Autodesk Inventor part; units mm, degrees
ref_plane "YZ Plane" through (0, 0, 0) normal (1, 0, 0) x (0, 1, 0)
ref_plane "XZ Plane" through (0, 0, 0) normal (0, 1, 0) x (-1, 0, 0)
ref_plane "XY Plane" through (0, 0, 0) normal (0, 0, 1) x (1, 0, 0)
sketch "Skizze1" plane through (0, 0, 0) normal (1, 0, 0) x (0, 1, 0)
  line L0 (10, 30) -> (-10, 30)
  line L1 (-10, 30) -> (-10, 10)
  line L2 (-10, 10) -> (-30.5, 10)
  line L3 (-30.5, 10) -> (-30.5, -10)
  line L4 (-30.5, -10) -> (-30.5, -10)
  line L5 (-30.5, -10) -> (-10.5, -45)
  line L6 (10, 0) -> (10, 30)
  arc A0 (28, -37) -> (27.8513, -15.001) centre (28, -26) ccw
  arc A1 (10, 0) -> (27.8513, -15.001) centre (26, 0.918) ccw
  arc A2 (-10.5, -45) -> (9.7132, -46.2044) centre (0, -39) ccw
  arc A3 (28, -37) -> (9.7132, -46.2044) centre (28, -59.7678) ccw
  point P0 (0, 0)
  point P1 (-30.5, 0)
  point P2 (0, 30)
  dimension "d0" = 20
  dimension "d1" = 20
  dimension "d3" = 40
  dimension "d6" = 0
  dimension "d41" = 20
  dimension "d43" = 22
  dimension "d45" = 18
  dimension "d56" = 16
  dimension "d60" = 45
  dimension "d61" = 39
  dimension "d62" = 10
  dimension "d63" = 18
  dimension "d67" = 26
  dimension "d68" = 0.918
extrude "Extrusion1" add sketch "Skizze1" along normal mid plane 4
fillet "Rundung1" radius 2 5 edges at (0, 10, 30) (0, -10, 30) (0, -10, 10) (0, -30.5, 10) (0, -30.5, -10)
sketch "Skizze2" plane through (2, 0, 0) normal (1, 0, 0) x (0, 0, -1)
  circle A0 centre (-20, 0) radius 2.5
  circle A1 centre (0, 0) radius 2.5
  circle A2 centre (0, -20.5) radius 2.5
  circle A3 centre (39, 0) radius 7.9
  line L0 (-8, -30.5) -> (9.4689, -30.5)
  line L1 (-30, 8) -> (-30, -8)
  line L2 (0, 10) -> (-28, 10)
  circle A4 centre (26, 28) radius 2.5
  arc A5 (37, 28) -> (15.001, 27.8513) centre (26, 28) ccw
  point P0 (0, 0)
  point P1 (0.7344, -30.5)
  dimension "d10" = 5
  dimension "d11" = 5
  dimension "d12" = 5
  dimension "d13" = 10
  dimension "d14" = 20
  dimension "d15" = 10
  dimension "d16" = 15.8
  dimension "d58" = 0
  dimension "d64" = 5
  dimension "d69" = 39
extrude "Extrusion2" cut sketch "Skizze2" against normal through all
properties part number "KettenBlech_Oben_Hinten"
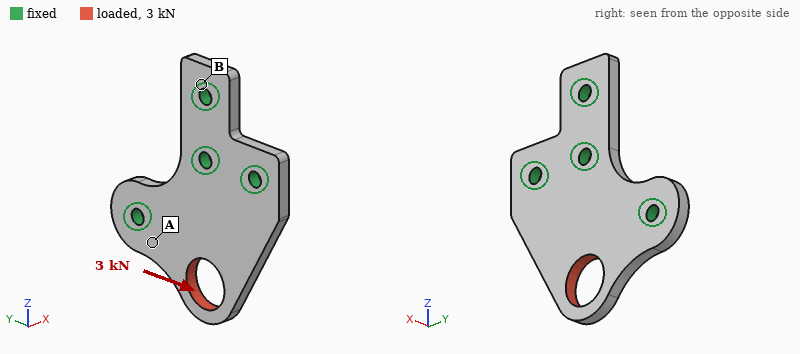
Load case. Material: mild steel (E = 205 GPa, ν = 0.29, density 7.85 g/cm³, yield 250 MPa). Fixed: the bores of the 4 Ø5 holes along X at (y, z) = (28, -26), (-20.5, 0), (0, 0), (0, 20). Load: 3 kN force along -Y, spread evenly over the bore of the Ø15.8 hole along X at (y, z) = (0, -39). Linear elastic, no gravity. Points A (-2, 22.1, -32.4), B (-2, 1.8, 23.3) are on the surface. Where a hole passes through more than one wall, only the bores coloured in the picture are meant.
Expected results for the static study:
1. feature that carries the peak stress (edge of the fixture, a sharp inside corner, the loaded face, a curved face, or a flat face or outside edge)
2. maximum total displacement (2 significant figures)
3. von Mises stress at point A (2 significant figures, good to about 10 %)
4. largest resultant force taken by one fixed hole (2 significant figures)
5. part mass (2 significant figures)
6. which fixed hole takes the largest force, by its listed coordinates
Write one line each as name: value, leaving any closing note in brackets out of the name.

feature that carries the peak stress: the loaded face
maximum total displacement: 17 µm
von Mises stress at point A: 44 MPa
largest resultant force taken by one fixed hole: 2.5 kN
part mass: 87 g
which fixed hole takes the largest force, by its listed coordinates: (28, -26)
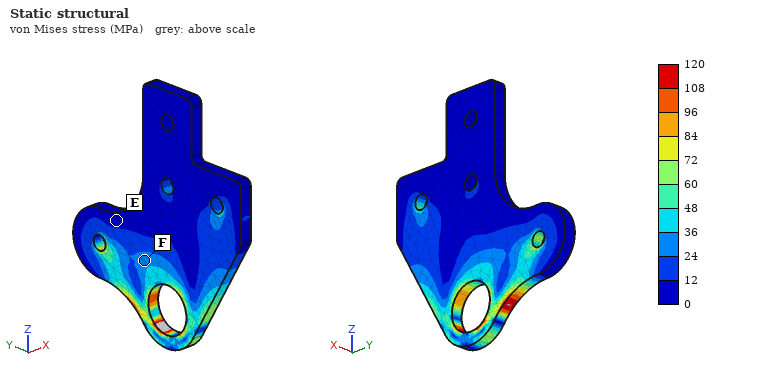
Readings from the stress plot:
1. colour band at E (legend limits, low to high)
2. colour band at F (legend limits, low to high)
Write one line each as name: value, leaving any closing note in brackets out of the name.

colour band at E: 0 to 12 MPa
colour band at F: 24 to 36 MPa
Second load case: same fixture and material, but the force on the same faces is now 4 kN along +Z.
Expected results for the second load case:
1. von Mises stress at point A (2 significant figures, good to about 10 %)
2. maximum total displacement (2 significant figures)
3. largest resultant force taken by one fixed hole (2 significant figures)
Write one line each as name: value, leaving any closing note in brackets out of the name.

von Mises stress at point A: 17 MPa
maximum total displacement: 11 µm
largest resultant force taken by one fixed hole: 1.6 kN
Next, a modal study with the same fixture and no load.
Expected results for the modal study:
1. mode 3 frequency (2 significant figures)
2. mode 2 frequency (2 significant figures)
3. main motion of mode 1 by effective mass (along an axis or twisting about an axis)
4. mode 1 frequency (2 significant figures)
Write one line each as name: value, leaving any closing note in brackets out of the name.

mode 3 frequency: 11 kHz
mode 2 frequency: 8100 Hz
main motion of mode 1 by effective mass: along X
mode 1 frequency: 3400 Hz
